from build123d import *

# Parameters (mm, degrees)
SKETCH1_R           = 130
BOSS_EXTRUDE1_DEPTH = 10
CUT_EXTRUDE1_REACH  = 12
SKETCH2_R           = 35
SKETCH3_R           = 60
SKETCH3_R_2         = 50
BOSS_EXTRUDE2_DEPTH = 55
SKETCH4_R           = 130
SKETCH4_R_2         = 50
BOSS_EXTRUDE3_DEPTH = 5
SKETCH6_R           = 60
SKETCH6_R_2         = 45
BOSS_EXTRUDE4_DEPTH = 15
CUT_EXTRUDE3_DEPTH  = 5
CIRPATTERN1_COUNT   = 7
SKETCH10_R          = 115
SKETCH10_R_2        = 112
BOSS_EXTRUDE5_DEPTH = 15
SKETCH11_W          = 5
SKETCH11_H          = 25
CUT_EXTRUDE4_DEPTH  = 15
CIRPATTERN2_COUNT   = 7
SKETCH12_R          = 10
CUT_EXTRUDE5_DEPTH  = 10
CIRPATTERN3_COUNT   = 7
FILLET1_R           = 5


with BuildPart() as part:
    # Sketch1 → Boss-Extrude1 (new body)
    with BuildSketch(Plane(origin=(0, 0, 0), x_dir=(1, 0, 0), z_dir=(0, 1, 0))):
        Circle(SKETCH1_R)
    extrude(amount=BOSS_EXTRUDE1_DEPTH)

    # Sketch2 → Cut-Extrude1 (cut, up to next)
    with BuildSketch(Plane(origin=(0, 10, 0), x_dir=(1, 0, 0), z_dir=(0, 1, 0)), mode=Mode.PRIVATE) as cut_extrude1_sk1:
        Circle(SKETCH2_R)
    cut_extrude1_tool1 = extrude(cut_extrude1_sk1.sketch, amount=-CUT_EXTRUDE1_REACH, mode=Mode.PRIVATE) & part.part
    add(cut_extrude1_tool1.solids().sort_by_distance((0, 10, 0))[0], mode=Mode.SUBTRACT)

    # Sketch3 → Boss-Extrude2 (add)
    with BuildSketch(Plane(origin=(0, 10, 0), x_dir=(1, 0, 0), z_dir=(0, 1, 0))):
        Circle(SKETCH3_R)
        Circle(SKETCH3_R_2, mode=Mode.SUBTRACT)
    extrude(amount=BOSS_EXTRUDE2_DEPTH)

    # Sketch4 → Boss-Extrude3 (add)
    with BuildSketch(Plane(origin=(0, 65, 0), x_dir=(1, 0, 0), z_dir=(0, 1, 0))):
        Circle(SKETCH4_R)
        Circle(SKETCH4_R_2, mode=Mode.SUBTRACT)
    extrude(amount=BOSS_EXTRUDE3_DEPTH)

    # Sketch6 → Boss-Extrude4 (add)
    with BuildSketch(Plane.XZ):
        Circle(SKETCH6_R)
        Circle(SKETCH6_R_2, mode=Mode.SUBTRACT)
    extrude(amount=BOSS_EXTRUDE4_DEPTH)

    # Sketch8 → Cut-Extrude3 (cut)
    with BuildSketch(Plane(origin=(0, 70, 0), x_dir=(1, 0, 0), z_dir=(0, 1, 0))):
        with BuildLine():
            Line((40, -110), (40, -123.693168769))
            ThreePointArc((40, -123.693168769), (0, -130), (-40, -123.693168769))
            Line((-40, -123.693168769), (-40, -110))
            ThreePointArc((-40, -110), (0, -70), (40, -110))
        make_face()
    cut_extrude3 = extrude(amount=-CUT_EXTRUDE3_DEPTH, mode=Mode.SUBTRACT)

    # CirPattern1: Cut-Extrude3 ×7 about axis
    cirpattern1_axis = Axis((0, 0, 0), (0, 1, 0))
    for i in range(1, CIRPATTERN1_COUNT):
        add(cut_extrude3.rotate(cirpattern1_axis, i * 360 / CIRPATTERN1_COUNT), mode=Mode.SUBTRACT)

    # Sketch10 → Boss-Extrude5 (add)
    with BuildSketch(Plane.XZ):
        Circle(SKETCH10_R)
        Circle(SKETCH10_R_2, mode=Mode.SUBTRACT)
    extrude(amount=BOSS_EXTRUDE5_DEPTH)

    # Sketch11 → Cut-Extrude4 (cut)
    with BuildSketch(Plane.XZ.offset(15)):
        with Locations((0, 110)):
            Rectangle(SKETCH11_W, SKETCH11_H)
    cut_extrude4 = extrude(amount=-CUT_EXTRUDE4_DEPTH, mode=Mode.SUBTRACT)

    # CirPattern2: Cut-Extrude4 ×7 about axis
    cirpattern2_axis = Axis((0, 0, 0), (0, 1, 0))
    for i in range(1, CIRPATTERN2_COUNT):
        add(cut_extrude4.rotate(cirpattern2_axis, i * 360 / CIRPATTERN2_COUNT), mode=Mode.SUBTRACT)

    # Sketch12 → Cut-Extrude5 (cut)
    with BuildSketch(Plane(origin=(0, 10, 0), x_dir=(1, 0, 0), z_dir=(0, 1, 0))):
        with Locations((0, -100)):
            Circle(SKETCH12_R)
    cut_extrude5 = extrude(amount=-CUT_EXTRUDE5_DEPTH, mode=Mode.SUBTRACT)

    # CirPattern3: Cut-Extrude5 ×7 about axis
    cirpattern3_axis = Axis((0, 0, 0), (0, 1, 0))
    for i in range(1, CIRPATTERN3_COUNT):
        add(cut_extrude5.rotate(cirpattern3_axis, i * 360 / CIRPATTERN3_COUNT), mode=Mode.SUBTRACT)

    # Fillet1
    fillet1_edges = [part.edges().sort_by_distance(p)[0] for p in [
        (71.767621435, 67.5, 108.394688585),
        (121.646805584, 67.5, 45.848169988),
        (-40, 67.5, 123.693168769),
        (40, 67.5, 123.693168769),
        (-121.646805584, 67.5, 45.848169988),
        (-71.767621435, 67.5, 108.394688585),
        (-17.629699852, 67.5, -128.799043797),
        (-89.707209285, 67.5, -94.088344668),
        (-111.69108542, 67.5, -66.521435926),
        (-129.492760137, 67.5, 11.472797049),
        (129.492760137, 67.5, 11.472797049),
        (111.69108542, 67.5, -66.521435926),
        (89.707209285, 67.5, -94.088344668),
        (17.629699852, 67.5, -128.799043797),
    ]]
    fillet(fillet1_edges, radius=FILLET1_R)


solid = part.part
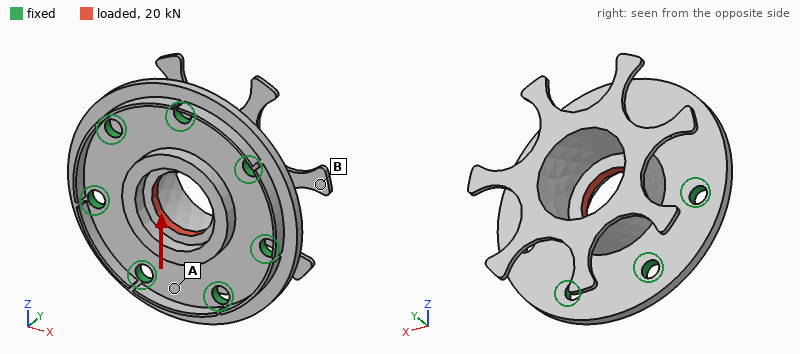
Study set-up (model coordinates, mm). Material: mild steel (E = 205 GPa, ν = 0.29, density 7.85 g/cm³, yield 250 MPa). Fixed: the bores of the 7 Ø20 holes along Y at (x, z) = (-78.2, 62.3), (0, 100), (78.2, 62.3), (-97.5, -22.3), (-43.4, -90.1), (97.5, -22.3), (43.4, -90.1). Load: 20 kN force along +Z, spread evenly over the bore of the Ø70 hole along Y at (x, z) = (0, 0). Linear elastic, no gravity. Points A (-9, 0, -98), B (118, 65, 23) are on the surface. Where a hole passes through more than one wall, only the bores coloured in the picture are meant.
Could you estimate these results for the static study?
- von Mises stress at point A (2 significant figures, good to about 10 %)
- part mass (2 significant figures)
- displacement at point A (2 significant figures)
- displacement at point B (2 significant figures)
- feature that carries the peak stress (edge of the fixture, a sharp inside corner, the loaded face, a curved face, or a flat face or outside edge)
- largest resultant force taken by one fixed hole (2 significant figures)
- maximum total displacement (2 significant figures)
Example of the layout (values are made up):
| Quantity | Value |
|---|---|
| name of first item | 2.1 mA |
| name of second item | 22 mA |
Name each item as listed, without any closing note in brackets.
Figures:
| Quantity | Value |
|---|---|
| von Mises stress at point A | 2.6 MPa |
| part mass | 6.7 kg |
| displacement at point A | 0.91 µm |
| displacement at point B | 1.4 µm |
| feature that carries the peak stress | a sharp inside corner |
| largest resultant force taken by one fixed hole | 4.4 kN |
| maximum total displacement | 2.6 µm |
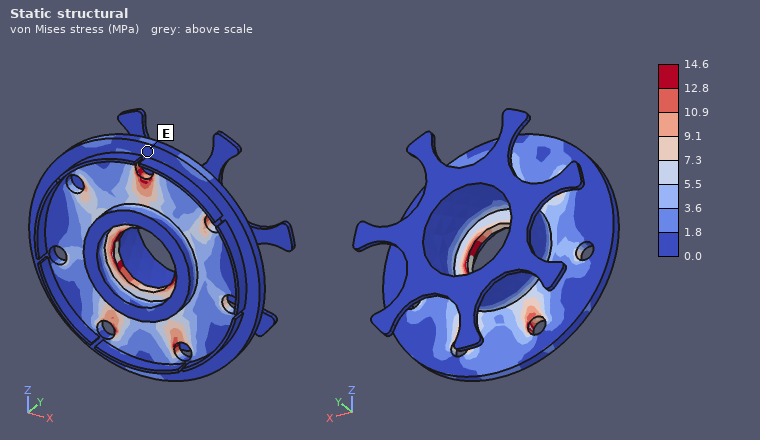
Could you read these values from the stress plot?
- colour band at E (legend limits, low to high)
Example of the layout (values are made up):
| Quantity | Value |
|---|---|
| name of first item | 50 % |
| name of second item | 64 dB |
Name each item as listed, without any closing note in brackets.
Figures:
| Quantity | Value |
|---|---|
| colour band at E | 0.0 to 1.8 MPa |
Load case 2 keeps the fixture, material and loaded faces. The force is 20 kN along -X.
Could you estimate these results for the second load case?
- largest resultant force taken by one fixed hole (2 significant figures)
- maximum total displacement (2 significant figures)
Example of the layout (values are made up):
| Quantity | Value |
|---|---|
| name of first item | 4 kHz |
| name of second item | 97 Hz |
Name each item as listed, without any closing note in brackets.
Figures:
| Quantity | Value |
|---|---|
| largest resultant force taken by one fixed hole | 4.3 kN |
| maximum total displacement | 2.7 µm |
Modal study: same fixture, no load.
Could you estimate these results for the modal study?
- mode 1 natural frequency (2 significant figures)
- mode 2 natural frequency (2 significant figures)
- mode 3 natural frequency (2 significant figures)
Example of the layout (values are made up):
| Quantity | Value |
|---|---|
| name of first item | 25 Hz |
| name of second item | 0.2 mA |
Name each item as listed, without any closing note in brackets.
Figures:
| Quantity | Value |
|---|---|
| mode 1 natural frequency | 890 Hz |
| mode 2 natural frequency | 900 Hz |
| mode 3 natural frequency | 910 Hz |
